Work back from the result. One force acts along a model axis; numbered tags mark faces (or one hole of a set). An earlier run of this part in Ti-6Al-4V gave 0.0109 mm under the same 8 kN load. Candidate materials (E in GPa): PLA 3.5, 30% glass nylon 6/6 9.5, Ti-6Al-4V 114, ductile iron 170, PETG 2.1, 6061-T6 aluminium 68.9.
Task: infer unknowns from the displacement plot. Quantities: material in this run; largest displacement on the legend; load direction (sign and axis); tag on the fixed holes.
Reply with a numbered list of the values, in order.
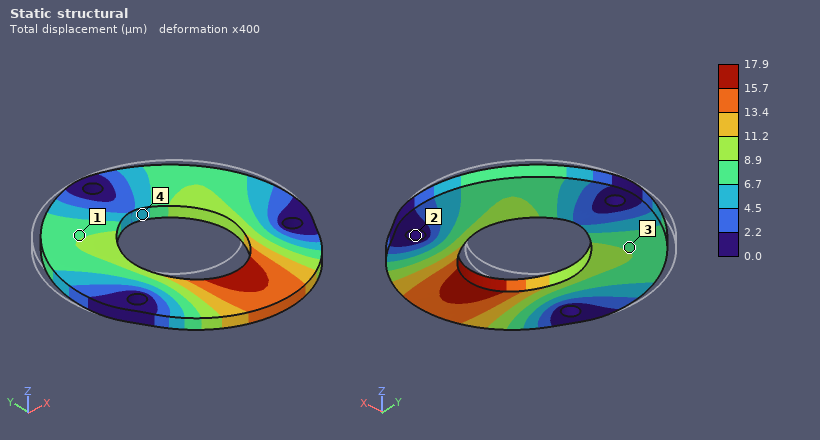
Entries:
1. 6061-T6 aluminium
2. 17.9 µm
3. -Y
4. 2
